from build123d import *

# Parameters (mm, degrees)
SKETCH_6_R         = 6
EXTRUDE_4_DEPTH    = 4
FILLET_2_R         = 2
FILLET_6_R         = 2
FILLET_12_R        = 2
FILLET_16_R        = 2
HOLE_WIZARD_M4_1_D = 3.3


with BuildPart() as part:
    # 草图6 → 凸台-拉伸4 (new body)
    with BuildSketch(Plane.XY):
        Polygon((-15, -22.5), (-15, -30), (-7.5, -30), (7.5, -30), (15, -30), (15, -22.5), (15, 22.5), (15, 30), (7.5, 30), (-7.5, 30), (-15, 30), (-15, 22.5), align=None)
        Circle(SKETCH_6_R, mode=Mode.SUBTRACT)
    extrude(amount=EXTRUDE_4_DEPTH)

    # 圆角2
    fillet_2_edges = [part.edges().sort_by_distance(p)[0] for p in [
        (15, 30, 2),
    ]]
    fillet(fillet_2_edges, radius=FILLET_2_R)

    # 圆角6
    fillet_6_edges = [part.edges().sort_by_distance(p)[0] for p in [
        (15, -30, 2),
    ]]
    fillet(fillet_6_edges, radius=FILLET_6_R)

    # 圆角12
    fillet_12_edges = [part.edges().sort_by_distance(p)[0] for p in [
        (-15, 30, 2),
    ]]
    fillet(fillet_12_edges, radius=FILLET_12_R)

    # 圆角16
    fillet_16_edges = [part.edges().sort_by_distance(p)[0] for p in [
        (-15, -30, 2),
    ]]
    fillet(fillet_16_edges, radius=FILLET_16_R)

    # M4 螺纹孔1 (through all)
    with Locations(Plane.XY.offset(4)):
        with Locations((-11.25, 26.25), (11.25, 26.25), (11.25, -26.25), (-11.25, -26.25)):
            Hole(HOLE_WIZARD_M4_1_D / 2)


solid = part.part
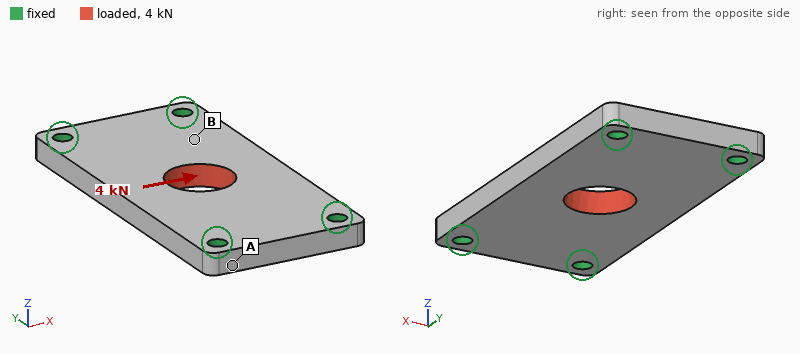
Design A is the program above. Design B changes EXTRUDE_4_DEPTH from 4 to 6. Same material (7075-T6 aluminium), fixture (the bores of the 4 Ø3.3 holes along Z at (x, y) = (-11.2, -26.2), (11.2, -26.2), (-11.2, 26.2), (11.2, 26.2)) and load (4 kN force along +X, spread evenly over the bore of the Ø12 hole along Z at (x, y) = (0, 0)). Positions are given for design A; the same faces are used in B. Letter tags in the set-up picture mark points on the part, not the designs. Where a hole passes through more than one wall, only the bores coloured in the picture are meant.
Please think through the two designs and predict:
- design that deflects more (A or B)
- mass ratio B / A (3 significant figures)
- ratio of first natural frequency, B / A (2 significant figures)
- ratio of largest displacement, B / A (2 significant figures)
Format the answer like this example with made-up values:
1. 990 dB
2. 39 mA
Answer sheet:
1. A
2. 1.50
3. 1.4
4. 0.67
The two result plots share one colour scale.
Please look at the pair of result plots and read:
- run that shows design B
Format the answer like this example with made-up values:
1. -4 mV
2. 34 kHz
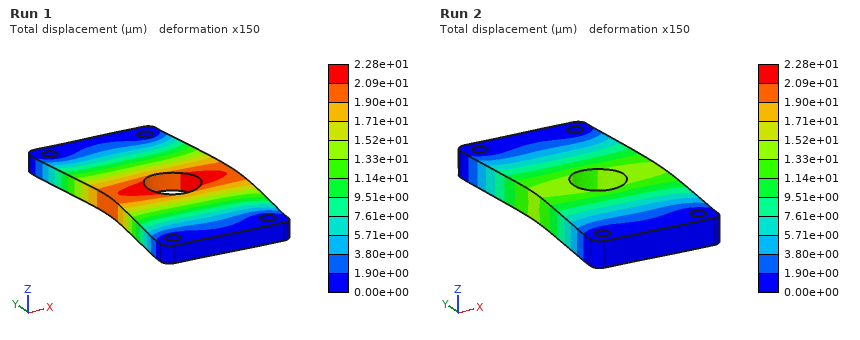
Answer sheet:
1. Run 2
